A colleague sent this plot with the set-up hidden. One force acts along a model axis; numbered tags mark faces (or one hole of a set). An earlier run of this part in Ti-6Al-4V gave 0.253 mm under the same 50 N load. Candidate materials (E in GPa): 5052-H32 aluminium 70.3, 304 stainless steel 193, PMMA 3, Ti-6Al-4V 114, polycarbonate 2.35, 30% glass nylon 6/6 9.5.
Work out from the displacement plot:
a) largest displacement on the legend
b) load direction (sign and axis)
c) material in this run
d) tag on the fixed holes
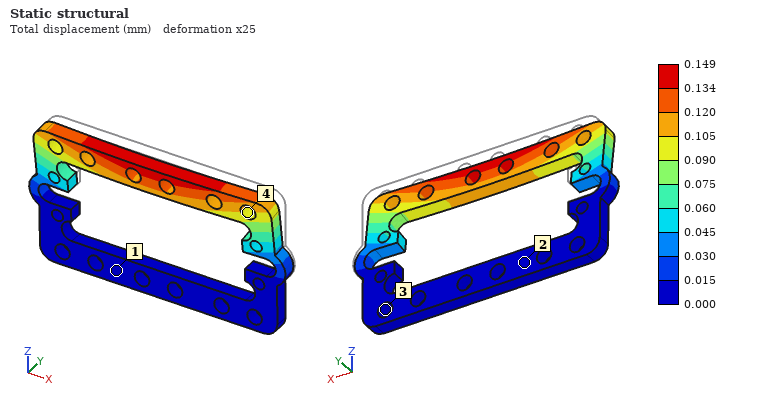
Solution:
0.149 mm
-Y
304 stainless steel
3
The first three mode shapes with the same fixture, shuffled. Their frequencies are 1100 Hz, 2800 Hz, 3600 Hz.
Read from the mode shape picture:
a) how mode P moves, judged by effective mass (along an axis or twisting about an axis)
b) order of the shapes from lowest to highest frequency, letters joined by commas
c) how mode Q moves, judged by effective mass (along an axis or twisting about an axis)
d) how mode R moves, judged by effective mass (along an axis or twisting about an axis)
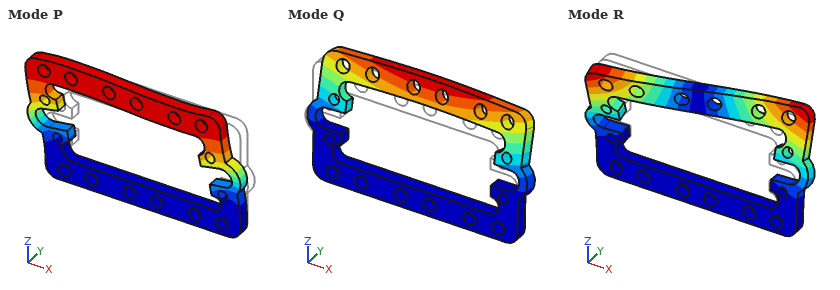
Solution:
along X
Q, R, P
along Y
twisting about Z
